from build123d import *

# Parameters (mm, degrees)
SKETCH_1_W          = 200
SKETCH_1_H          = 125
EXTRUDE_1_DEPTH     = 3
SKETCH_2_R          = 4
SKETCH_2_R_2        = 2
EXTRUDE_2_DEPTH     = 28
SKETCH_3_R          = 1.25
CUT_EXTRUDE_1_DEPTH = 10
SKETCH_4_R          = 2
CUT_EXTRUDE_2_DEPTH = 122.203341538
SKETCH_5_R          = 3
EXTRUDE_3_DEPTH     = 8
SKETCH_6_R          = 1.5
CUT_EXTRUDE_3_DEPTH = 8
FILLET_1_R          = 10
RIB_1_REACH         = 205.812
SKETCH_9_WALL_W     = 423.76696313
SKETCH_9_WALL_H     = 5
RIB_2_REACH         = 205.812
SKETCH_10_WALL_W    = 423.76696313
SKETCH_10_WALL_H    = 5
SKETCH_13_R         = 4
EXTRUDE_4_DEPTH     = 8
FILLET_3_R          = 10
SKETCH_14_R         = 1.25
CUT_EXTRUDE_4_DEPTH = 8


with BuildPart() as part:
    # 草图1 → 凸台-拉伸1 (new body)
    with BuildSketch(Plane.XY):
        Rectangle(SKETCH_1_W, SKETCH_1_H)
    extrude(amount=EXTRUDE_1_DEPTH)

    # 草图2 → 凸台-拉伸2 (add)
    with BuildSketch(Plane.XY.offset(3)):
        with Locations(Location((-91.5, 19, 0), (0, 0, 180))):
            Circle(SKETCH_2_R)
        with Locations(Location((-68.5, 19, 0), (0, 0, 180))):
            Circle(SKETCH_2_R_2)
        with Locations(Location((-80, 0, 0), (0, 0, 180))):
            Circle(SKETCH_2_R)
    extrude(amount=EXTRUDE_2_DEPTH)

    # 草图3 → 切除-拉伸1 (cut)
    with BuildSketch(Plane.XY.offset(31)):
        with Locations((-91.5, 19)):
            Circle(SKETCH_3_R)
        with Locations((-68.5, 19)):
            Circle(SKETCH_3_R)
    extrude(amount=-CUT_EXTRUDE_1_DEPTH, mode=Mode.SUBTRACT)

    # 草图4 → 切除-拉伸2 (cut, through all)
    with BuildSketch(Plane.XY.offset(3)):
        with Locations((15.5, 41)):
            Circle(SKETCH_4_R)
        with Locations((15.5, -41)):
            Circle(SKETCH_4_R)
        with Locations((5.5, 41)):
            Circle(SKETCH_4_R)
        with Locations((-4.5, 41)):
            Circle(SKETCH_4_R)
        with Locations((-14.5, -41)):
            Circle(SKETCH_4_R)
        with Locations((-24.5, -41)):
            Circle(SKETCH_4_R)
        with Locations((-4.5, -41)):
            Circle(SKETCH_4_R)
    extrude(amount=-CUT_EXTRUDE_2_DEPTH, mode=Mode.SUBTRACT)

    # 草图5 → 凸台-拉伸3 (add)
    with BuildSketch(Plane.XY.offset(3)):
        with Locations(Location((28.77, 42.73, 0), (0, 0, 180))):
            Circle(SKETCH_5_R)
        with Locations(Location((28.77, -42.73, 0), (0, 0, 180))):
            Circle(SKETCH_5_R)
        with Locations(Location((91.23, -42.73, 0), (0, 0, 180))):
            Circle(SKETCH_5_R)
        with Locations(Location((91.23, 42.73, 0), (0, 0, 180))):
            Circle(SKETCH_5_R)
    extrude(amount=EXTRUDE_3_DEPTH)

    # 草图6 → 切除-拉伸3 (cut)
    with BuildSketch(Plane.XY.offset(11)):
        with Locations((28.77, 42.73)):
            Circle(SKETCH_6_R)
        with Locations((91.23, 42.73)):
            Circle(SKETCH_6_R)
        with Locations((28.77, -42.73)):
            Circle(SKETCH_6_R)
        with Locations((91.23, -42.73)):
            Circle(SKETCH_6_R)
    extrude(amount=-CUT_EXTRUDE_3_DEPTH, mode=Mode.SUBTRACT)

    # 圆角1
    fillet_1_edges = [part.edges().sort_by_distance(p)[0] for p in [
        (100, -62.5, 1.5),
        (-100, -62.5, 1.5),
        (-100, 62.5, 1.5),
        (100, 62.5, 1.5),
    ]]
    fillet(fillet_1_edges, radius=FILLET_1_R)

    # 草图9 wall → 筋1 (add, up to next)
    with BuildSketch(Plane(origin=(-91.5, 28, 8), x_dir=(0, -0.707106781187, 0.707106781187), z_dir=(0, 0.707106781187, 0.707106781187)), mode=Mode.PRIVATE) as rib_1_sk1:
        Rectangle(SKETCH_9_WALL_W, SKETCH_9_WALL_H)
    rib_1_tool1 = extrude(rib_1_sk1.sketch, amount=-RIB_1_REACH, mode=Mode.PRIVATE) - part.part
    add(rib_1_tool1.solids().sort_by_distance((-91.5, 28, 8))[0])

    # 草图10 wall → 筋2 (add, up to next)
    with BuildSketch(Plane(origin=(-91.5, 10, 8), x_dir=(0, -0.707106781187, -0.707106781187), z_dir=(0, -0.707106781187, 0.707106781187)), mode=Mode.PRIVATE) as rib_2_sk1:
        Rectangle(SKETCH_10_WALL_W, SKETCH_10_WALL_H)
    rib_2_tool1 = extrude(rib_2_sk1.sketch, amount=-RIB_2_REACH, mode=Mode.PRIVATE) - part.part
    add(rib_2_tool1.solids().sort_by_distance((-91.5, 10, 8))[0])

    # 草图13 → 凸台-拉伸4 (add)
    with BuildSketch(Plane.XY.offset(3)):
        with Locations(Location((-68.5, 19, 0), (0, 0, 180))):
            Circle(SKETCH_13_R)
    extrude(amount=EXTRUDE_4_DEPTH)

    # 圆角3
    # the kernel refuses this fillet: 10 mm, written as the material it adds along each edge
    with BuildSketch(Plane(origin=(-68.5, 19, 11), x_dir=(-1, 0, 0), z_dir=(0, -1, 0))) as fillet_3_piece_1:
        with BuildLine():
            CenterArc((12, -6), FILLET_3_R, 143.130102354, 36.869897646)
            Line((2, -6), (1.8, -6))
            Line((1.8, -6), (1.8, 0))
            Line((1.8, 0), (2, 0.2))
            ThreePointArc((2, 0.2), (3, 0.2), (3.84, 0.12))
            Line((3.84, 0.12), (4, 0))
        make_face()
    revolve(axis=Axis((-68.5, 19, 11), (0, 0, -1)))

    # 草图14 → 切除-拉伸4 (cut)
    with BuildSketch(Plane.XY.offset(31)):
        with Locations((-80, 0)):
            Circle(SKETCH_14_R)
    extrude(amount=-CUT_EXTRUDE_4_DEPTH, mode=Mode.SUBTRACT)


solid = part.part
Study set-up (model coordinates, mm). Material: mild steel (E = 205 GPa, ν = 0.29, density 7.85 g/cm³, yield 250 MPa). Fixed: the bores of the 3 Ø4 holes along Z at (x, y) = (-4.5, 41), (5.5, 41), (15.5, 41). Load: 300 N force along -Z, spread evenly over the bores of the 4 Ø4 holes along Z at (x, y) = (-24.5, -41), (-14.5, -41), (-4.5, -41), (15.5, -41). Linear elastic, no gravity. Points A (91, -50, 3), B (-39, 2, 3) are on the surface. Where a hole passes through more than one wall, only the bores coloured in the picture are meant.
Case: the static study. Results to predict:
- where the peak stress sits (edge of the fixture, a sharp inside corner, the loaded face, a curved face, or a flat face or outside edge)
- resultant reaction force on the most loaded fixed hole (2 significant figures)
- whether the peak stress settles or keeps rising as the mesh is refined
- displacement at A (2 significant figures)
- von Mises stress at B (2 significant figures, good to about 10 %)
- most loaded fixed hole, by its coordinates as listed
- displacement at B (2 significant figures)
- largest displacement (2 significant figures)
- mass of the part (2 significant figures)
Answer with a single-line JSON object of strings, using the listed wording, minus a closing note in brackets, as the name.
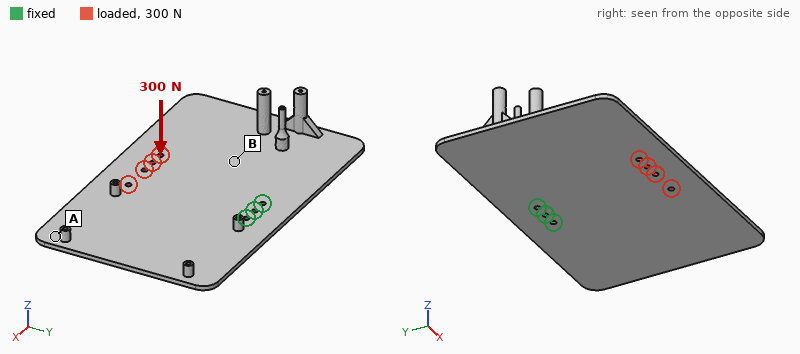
{"where the peak stress sits": "edge of the fixture", "resultant reaction force on the most loaded fixed hole": "200 N", "whether the peak stress settles or keeps rising as the mesh is refined": "keeps rising", "displacement at A": "0.92 mm", "von Mises stress at B": "44 MPa", "most loaded fixed hole, by its coordinates as listed": "(-4.5, 41)", "displacement at B": "0.48 mm", "largest displacement": "1.6 mm", "mass of the part": "620 g"}
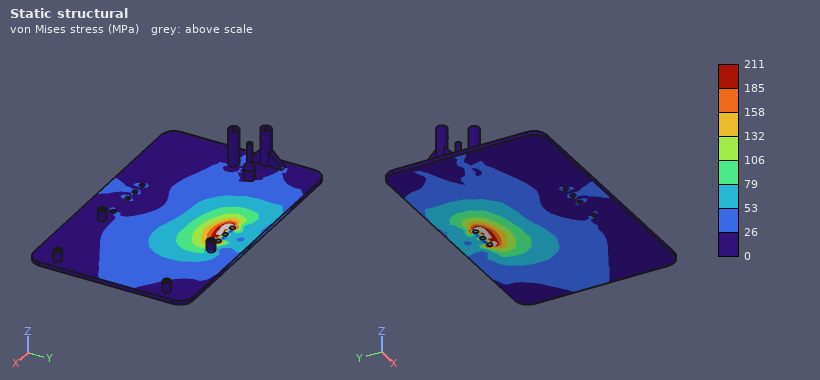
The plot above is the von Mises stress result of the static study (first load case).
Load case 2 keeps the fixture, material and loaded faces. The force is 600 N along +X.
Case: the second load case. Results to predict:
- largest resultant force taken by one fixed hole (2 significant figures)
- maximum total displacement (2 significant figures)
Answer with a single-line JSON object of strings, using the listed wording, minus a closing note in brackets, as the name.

{"largest resultant force taken by one fixed hole": "2.1 kN", "maximum total displacement": "42 µm"}
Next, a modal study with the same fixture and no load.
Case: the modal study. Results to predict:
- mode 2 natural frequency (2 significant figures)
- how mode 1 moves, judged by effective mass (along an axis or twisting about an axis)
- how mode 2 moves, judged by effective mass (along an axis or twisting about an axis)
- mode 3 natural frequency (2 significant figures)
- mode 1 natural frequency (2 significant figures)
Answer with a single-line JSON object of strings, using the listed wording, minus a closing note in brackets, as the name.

{"mode 2 natural frequency": "170 Hz", "how mode 1 moves, judged by effective mass": "along Z", "how mode 2 moves, judged by effective mass": "along Z", "mode 3 natural frequency": "310 Hz", "mode 1 natural frequency": "150 Hz"}
